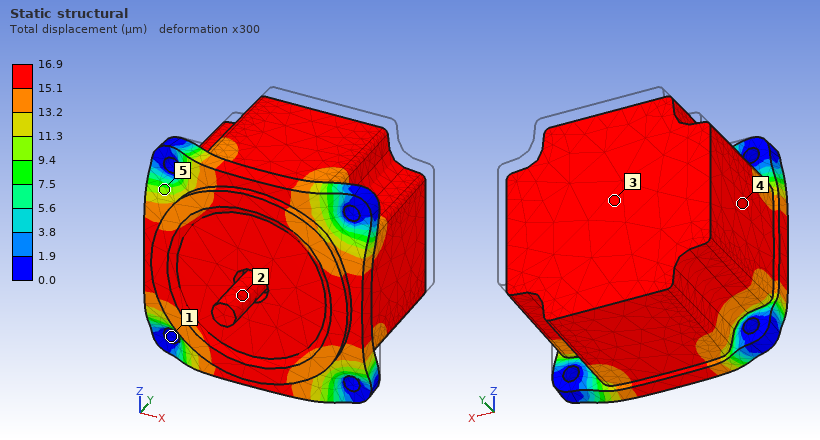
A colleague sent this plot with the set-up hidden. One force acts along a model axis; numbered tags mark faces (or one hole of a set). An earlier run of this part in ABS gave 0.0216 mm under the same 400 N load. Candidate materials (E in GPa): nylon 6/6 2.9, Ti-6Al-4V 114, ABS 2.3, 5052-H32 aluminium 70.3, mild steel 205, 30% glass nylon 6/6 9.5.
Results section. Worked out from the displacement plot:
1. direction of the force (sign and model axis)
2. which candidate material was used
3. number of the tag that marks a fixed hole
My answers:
-Y
nylon 6/6
1
